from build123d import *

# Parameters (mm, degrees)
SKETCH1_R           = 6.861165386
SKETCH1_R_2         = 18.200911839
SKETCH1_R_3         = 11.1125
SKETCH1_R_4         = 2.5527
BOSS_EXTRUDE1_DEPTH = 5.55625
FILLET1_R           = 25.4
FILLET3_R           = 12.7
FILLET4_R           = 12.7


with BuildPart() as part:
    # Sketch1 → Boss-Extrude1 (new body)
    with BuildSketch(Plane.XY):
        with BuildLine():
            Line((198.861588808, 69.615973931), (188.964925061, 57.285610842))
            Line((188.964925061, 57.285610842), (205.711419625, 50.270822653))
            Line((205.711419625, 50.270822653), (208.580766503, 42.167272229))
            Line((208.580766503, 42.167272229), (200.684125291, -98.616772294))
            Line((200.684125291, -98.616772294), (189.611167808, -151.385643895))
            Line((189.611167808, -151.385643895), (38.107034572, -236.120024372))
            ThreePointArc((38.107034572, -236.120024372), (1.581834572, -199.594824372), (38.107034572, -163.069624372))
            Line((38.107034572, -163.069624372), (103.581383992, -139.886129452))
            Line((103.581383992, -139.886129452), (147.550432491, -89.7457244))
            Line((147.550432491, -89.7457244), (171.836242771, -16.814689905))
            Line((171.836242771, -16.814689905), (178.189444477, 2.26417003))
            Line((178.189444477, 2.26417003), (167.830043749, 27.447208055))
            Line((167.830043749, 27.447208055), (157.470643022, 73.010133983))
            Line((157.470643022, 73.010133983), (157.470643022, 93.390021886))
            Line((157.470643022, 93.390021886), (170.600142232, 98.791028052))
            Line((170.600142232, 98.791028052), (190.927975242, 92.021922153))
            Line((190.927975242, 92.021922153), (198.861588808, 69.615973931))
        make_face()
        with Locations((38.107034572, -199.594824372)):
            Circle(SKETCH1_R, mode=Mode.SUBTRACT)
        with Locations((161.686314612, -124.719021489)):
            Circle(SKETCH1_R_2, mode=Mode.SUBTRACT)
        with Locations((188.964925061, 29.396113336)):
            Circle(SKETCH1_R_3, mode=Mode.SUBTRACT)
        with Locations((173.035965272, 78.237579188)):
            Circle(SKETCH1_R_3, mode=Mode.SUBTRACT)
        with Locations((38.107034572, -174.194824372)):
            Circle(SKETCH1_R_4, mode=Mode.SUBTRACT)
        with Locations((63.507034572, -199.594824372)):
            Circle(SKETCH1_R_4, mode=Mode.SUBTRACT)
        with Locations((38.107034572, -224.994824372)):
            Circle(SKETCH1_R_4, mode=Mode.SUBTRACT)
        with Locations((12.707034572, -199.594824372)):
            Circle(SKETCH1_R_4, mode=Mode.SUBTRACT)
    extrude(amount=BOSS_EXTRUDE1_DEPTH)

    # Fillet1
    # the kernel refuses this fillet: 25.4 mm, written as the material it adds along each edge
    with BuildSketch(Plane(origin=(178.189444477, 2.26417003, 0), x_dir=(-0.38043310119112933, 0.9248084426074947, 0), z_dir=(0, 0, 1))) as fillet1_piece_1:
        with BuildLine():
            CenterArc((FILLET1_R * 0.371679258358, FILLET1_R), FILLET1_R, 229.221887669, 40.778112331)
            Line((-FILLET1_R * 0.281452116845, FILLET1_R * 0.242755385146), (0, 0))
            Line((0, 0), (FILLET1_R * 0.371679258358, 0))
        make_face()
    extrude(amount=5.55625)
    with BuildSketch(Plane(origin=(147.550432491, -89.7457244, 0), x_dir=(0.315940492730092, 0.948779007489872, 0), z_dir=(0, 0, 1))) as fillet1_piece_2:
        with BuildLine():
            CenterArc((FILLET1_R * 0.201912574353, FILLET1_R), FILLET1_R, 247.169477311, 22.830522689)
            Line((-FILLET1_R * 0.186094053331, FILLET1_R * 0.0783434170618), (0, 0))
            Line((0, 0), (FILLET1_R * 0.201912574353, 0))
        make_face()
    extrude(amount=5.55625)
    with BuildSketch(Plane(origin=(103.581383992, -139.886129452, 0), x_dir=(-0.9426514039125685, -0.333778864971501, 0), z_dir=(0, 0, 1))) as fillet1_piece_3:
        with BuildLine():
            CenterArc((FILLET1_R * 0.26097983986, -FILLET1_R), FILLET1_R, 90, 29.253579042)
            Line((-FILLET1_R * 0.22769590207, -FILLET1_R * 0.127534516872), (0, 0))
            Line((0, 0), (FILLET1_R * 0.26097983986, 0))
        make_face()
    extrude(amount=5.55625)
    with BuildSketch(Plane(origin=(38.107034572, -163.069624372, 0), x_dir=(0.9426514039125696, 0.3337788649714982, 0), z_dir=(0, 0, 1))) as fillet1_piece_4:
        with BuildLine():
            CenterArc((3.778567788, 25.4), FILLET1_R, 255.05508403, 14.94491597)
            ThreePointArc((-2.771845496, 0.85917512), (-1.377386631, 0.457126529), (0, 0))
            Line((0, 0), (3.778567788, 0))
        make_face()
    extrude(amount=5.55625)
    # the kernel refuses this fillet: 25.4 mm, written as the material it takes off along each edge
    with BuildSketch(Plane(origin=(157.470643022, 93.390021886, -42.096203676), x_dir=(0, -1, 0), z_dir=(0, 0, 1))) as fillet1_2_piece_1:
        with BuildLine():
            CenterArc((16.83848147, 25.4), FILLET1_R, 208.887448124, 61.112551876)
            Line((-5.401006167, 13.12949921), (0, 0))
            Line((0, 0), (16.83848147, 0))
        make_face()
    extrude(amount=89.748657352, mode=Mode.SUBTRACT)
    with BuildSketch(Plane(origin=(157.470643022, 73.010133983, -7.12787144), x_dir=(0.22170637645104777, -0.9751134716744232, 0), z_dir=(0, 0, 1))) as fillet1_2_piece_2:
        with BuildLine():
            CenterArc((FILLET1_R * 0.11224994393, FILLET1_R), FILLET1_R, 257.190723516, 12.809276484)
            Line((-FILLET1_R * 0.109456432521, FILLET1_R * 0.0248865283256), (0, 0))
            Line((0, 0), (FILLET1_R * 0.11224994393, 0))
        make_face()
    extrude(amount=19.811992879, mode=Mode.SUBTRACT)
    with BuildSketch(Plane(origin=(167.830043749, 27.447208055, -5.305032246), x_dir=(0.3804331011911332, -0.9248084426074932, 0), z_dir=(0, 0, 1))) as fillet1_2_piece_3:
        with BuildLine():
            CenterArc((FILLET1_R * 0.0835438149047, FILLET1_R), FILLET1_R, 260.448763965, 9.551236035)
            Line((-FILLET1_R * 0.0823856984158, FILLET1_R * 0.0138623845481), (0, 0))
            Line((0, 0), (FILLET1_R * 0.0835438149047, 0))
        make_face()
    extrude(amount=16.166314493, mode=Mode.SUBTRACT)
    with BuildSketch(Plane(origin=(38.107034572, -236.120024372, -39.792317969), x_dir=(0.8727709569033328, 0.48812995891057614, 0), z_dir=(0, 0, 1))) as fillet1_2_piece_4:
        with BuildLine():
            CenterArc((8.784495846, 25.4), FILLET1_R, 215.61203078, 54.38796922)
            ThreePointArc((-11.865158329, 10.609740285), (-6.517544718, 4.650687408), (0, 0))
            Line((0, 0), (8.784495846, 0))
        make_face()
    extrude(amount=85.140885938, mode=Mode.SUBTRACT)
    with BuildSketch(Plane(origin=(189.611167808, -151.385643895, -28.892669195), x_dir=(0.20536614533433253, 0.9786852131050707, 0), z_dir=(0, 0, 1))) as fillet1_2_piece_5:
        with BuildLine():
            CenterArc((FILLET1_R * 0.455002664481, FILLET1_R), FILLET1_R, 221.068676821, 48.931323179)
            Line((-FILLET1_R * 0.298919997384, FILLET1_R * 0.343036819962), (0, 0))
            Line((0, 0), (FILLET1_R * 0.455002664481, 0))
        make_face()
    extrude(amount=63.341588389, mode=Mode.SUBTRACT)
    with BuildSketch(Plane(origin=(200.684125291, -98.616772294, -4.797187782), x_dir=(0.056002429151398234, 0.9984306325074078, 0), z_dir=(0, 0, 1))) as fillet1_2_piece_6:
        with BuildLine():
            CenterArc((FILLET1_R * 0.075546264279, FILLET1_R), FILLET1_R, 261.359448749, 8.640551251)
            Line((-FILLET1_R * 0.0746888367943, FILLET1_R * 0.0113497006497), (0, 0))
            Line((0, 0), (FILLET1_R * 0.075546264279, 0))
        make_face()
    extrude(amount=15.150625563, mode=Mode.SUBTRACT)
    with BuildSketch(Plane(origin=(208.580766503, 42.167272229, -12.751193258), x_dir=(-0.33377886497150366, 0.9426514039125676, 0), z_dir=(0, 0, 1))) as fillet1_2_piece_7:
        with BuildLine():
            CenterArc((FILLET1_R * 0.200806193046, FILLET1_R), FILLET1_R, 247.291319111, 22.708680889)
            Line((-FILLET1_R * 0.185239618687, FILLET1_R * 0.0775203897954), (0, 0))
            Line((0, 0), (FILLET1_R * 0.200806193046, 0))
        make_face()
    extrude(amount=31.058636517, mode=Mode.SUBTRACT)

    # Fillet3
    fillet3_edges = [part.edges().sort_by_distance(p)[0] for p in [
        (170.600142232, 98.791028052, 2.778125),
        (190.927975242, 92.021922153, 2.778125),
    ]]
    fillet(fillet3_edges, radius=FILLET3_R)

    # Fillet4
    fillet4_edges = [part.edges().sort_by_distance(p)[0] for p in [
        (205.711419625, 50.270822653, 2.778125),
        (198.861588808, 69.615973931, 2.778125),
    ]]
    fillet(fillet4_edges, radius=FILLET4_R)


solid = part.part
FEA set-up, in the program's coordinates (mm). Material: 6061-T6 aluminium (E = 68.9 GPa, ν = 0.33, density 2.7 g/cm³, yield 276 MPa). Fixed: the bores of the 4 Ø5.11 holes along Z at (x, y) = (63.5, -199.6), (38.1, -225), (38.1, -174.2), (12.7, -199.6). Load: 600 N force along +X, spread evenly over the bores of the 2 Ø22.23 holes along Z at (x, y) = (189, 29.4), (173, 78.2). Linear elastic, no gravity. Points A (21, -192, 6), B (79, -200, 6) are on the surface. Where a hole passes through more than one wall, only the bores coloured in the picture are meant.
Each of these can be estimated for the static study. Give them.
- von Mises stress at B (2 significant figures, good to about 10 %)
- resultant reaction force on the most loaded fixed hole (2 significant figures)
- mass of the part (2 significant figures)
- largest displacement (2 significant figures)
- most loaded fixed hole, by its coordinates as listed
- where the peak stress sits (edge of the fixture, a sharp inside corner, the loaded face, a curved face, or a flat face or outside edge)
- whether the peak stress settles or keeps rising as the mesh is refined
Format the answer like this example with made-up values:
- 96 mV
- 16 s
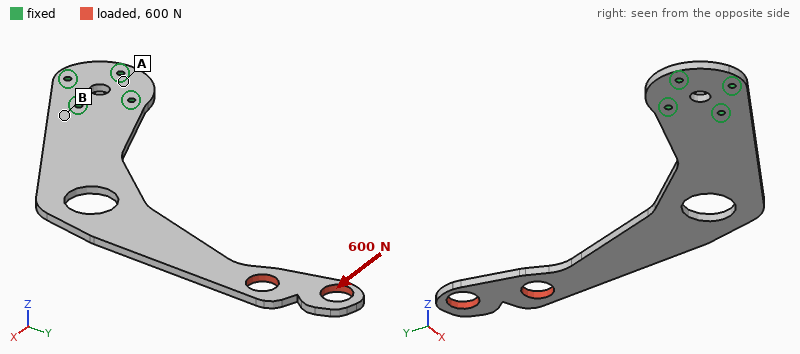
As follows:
- 26 MPa
- 3.2 kN
- 270 g
- 1.4 mm
- (38.1, -174.2)
- edge of the fixture
- keeps rising
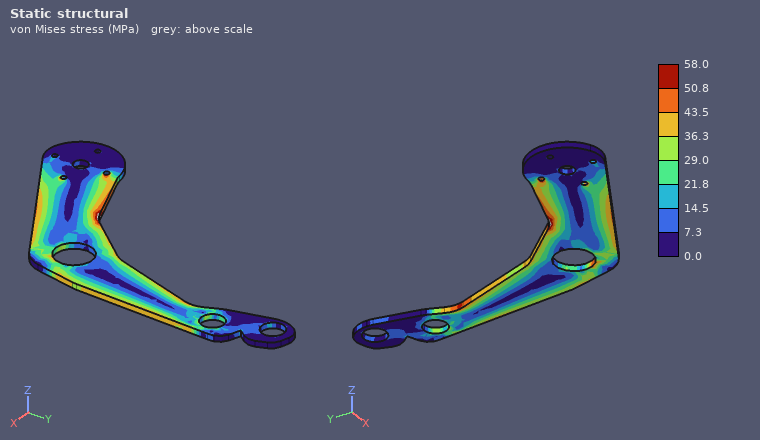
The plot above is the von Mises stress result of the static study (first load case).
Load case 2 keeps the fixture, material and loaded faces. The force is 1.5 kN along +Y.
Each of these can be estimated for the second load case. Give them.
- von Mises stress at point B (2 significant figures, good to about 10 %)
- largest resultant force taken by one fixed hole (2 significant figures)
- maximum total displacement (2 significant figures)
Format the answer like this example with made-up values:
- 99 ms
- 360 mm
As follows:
- 33 MPa
- 3.7 kN
- 0.71 mm
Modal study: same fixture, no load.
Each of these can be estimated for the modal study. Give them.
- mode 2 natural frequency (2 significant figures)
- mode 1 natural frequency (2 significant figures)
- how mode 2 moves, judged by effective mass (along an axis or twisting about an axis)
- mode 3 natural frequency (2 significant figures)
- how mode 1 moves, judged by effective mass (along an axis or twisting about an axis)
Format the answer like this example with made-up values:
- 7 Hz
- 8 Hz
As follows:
- 200 Hz
- 54 Hz
- along Z
- 490 Hz
- along Z
